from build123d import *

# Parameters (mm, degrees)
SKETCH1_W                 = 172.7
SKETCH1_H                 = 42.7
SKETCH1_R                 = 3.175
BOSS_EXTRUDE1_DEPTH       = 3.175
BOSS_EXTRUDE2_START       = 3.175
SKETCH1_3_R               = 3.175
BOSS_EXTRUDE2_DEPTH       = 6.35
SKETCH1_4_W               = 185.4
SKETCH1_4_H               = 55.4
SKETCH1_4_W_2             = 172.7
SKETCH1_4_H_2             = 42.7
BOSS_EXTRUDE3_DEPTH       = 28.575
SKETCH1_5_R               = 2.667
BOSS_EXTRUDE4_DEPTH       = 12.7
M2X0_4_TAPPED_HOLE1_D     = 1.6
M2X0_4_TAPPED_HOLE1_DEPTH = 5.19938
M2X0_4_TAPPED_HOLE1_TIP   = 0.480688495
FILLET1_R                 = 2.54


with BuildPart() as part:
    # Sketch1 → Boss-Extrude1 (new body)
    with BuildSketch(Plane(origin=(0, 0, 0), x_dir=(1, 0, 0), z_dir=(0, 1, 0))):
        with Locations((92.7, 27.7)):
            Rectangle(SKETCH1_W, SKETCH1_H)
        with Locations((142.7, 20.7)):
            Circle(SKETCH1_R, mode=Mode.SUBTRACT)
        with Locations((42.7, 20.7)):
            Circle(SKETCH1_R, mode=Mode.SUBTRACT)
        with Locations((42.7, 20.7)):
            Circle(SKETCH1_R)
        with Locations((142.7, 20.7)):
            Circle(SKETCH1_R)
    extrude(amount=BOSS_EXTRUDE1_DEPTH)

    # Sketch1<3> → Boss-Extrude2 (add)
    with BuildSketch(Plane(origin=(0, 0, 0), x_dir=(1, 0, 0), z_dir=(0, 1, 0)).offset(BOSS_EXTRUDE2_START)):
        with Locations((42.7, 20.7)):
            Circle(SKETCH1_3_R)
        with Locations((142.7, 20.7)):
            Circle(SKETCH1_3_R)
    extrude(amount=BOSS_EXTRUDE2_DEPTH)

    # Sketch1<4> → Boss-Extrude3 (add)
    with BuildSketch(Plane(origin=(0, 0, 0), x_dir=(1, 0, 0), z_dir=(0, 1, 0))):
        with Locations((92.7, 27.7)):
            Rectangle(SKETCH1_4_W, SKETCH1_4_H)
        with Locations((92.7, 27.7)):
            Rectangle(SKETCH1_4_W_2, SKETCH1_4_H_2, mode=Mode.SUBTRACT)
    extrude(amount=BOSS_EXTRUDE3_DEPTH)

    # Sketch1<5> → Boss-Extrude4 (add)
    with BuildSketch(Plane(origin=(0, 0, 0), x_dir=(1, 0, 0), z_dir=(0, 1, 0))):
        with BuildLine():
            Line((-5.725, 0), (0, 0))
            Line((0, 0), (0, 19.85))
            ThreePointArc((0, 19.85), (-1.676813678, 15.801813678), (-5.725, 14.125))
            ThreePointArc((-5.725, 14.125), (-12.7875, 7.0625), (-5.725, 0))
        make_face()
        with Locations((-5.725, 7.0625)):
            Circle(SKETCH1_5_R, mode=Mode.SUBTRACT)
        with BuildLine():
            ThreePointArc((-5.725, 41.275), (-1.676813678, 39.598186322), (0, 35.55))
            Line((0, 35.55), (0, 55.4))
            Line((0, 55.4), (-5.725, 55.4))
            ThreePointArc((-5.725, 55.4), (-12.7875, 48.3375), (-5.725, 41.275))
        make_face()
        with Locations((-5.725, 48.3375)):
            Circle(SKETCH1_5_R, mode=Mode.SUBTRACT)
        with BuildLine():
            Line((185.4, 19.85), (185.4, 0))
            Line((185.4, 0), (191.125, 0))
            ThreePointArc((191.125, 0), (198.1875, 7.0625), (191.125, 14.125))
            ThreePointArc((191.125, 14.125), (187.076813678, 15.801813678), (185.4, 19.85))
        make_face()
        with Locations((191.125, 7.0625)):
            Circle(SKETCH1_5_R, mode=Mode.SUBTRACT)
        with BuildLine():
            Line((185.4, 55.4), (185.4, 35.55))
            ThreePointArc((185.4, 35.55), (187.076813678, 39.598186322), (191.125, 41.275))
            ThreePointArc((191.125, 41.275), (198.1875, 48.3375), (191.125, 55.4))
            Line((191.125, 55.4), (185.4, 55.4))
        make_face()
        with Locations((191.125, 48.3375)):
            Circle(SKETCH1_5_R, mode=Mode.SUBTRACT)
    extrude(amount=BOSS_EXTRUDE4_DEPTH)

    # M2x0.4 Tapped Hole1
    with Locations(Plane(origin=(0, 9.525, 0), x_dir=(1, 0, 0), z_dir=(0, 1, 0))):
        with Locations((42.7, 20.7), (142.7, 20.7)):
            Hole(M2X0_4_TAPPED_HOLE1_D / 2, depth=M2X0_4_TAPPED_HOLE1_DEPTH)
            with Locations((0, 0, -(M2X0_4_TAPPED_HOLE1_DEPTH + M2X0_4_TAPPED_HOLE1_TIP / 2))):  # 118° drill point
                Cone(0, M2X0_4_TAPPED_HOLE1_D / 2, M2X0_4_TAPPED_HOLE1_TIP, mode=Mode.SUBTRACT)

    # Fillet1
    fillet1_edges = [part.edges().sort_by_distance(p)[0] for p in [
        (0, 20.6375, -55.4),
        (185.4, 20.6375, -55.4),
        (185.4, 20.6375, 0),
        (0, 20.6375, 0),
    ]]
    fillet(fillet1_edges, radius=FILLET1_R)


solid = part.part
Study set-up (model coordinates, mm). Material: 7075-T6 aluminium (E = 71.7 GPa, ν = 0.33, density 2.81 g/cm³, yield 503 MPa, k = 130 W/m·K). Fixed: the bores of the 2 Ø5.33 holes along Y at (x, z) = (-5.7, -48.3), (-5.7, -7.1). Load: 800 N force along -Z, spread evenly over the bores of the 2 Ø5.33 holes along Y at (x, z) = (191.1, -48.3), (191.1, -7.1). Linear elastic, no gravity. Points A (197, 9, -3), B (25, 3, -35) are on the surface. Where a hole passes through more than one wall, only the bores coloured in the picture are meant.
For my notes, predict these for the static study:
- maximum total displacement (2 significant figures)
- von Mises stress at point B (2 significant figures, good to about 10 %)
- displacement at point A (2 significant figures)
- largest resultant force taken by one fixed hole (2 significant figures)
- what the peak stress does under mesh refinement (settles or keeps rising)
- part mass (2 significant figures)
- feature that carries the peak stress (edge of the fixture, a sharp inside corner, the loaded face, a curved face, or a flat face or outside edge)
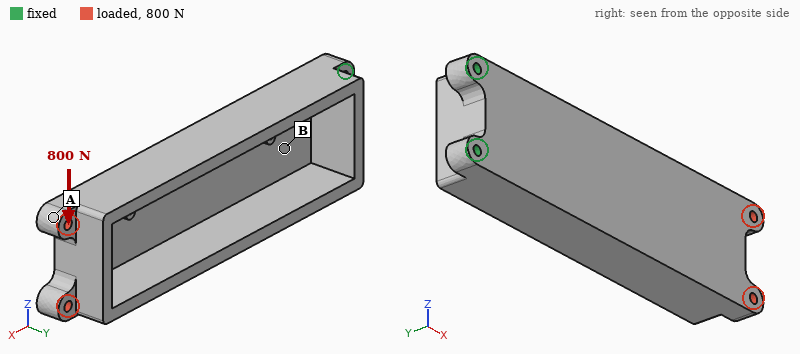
0.43 mm
14 MPa
0.34 mm
3.6 kN
keeps rising
320 g
edge of the fixture
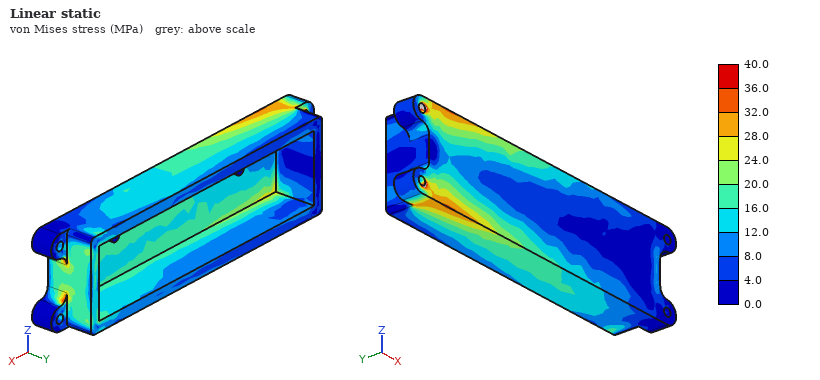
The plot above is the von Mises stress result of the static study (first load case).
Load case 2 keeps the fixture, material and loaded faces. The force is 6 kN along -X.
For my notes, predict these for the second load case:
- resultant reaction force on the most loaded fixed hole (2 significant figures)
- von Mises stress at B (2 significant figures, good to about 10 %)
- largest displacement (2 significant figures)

3.0 kN
15 MPa
0.16 mm
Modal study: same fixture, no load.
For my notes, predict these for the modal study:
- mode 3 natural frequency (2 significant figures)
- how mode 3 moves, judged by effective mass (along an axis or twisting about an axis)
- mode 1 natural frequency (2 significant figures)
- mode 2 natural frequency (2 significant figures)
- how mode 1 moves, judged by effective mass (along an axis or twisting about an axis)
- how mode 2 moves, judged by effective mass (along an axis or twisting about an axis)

1300 Hz
along Z
350 Hz
590 Hz
along Y
along Z
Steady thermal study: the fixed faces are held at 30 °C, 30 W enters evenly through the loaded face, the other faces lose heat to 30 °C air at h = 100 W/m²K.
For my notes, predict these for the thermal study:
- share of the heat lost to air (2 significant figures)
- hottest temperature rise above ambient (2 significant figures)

96 %
26 K
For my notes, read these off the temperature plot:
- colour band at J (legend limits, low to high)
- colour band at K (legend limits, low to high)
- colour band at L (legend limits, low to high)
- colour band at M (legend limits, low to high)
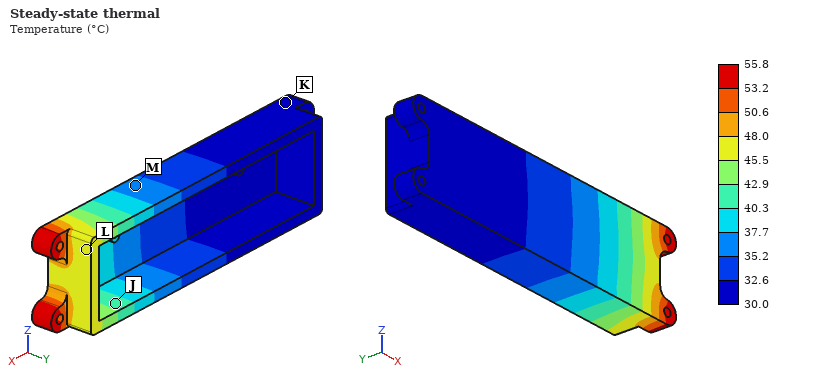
40.3 to 42.9 °C
30.0 to 32.6 °C
45.5 to 48.0 °C
35.2 to 37.7 °C
